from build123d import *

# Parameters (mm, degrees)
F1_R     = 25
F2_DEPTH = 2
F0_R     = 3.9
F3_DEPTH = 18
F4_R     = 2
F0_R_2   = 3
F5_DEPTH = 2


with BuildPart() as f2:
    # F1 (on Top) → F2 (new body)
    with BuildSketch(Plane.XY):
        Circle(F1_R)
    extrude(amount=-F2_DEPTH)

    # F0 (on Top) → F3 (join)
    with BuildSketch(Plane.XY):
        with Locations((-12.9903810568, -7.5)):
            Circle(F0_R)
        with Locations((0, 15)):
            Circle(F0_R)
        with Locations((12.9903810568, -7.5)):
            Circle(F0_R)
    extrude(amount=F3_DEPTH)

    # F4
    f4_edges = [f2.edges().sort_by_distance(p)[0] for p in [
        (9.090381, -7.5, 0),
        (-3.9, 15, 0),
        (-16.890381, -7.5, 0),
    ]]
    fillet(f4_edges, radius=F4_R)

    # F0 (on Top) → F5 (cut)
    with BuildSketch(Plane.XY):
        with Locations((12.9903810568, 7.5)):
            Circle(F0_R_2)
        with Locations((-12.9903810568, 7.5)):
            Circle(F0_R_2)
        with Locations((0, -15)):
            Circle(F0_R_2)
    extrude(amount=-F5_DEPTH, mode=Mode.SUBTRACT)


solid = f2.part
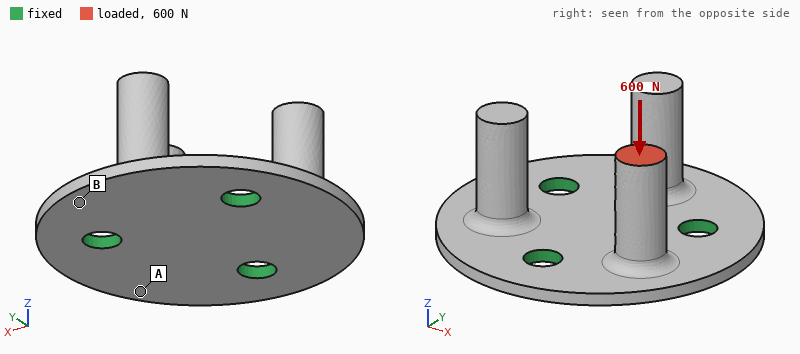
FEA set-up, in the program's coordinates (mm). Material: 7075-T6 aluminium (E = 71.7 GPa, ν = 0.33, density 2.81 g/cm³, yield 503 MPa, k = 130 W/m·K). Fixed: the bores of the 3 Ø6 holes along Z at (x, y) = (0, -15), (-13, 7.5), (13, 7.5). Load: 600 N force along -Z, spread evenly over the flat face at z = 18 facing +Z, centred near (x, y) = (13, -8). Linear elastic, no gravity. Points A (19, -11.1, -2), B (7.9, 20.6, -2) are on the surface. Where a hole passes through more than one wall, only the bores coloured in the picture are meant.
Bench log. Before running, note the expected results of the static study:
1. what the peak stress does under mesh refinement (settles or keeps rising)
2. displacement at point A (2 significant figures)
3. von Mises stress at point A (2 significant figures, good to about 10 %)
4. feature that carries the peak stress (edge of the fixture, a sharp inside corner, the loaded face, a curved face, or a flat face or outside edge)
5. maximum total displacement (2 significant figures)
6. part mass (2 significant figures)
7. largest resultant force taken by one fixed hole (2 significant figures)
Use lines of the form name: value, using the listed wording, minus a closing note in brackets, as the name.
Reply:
what the peak stress does under mesh refinement: keeps rising
displacement at point A: 0.12 mm
von Mises stress at point A: 44 MPa
feature that carries the peak stress: edge of the fixture
maximum total displacement: 0.18 mm
part mass: 18 g
largest resultant force taken by one fixed hole: 330 N
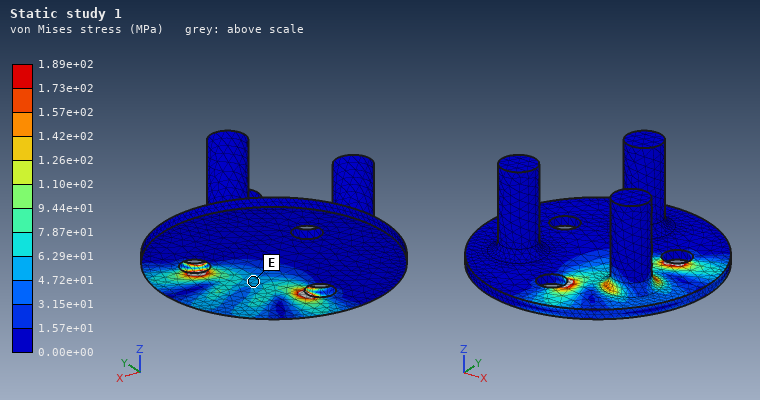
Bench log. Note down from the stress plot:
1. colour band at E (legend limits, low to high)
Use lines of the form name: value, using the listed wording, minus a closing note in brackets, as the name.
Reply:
colour band at E: 4.72e+01 to 6.29e+01 MPa
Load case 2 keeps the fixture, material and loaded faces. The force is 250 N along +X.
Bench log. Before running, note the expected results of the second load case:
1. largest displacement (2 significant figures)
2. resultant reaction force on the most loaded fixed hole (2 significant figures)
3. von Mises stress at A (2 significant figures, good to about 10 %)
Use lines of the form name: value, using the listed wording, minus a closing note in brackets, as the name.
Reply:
largest displacement: 0.30 mm
resultant reaction force on the most loaded fixed hole: 170 N
von Mises stress at A: 53 MPa
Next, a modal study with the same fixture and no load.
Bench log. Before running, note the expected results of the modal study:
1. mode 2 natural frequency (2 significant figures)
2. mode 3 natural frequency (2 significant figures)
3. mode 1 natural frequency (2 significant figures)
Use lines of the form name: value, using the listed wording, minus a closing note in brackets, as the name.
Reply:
mode 2 natural frequency: 4200 Hz
mode 3 natural frequency: 4200 Hz
mode 1 natural frequency: 4000 Hz
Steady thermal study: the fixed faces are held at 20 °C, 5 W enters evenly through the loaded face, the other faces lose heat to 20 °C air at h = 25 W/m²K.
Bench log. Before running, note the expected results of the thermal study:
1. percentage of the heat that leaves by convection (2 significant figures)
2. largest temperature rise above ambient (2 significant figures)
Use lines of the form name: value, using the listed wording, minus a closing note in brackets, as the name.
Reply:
percentage of the heat that leaves by convection: 5.4 %
largest temperature rise above ambient: 20 K
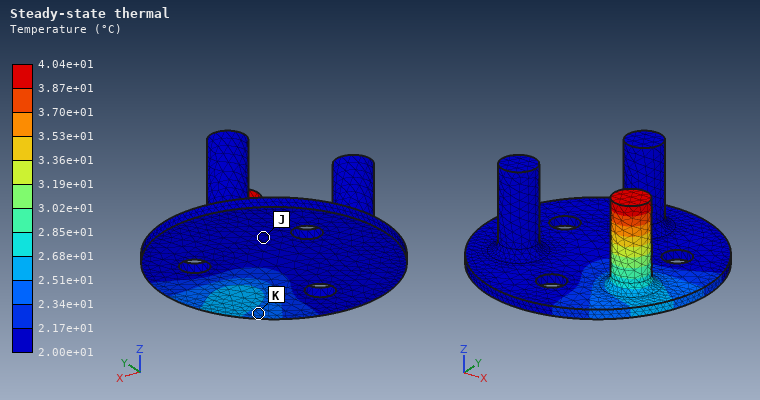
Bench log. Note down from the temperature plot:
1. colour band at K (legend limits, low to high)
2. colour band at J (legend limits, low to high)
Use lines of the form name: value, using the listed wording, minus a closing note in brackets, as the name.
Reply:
colour band at K: 2.34e+01 to 2.51e+01 °C
colour band at J: 2.00e+01 to 2.17e+01 °C
